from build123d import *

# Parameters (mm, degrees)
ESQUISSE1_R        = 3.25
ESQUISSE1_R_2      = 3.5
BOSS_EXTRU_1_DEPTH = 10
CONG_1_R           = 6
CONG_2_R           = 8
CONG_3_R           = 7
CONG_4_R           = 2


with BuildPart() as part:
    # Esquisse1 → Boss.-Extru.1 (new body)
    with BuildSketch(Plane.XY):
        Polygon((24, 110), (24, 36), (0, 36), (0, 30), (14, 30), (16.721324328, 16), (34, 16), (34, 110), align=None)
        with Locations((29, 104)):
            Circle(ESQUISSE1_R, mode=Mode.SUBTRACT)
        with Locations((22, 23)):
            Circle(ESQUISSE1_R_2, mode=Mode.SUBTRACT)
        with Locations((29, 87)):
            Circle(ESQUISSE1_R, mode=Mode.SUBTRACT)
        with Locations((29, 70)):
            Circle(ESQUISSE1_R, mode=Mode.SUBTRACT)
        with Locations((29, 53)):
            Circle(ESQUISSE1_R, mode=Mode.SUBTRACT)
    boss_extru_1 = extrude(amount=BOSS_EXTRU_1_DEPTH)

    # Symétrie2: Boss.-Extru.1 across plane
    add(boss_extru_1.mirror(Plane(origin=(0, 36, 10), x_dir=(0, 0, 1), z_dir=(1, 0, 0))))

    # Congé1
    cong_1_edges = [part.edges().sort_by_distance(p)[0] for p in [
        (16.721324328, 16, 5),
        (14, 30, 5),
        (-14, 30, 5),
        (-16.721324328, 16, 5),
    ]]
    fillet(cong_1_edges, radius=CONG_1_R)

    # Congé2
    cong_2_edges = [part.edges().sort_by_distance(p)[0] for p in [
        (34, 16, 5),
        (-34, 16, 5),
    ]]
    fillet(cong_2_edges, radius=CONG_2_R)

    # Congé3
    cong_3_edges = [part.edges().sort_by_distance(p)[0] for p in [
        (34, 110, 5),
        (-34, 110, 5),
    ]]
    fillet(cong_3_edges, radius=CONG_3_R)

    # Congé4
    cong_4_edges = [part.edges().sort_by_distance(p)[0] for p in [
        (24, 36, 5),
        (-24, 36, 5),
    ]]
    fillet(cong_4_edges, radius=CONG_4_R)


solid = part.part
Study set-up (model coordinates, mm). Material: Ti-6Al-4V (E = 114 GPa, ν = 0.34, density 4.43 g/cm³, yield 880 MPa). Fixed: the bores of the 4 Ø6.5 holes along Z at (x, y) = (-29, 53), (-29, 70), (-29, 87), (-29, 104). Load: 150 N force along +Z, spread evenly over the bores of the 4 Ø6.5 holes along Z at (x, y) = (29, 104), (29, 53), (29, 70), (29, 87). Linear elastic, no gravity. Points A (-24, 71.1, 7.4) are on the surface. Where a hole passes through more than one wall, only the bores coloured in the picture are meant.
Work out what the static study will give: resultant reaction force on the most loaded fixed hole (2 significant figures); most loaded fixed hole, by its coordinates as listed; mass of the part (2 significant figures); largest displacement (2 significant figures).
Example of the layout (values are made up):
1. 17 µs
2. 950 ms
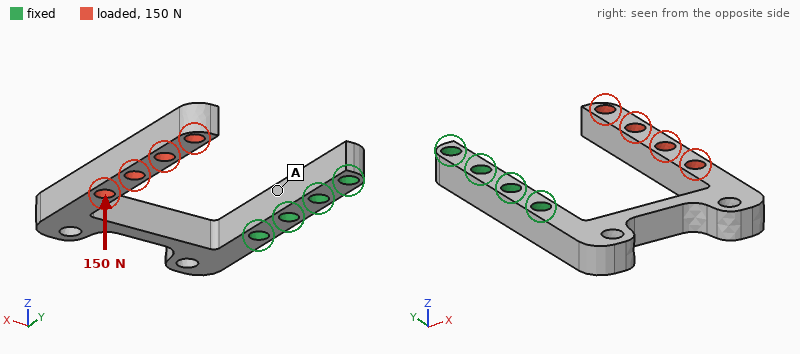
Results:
1. 150 N
2. (-29, 53)
3. 90 g
4. 1.3 mm
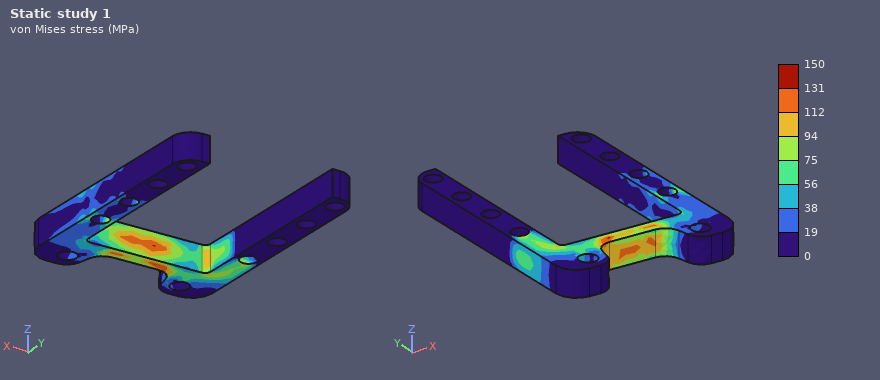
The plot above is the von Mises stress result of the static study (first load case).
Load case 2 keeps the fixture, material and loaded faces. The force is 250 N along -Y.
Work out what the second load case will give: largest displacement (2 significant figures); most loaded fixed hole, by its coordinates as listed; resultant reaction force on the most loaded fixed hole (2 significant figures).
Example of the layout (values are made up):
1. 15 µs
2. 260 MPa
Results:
1. 1.2 mm
2. (-29, 53)
3. 250 N
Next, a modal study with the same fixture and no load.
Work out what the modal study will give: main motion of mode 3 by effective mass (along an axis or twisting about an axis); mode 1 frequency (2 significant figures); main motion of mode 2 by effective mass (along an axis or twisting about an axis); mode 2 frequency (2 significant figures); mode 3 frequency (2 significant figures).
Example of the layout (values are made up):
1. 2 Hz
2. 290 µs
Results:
1. along Z
2. 390 Hz
3. along Z
4. 420 Hz
5. 910 Hz
